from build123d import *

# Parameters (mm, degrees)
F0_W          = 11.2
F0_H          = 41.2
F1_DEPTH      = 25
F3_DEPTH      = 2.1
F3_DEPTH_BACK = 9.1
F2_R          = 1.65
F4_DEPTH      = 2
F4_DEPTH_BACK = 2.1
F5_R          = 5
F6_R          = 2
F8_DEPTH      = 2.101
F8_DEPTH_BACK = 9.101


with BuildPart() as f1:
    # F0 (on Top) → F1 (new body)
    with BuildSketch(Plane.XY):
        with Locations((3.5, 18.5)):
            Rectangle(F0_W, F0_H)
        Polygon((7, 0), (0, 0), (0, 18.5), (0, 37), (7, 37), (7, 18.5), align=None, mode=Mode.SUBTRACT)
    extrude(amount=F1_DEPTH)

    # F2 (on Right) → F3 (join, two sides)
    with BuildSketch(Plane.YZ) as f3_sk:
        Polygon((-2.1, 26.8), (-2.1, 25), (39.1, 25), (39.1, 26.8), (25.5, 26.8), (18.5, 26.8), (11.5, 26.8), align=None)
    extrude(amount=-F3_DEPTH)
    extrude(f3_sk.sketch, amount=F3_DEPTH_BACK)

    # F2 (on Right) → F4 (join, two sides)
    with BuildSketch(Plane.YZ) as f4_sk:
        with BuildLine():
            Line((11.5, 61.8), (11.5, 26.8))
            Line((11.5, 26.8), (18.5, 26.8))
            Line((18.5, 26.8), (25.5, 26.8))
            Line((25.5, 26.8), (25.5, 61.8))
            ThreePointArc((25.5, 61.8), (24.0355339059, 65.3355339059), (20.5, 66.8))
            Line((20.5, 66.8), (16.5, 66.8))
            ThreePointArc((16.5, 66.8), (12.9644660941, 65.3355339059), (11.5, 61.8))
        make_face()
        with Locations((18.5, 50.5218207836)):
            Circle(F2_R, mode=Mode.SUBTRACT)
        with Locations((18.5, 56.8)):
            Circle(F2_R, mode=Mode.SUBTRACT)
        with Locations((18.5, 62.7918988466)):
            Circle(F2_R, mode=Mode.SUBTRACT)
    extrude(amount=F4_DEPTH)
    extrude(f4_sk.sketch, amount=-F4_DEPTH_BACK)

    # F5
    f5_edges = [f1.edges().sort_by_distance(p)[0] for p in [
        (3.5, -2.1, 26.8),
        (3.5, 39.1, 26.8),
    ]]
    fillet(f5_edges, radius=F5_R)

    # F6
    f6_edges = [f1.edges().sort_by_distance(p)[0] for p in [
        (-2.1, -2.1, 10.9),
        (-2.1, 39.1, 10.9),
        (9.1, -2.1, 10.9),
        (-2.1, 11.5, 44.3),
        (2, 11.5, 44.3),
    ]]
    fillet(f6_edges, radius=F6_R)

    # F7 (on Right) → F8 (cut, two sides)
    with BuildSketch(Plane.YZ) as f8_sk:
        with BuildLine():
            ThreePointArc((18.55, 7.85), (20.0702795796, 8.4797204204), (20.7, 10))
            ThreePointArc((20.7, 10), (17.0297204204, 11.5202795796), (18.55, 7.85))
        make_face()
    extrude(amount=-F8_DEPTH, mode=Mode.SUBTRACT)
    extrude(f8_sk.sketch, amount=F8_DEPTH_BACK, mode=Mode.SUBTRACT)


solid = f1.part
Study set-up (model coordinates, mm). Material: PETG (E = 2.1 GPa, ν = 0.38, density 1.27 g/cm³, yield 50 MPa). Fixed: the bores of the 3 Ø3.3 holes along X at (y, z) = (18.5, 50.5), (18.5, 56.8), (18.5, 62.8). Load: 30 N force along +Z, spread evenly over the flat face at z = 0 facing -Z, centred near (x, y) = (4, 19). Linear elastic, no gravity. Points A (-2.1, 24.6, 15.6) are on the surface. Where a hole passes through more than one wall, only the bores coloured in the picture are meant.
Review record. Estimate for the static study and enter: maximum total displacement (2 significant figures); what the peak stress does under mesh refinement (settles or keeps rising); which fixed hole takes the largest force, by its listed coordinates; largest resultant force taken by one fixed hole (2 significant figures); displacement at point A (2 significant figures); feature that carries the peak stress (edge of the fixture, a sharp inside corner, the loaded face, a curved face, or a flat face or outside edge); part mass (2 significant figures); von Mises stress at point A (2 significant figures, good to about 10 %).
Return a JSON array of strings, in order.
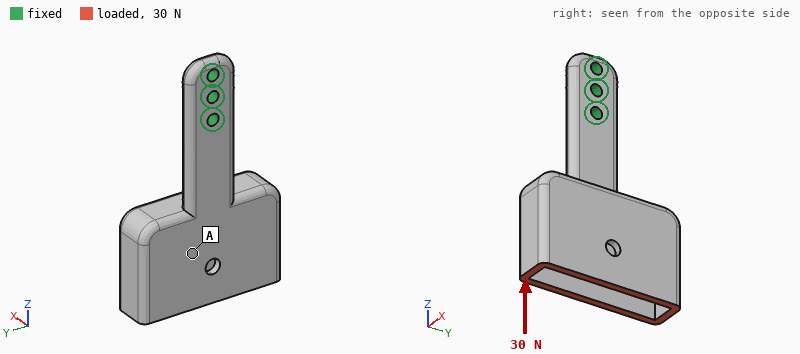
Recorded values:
["0.80 mm", "keeps rising", "(18.5, 50.5)", "24 N", "0.41 mm", "edge of the fixture", "9.6 g", "0.44 MPa"]
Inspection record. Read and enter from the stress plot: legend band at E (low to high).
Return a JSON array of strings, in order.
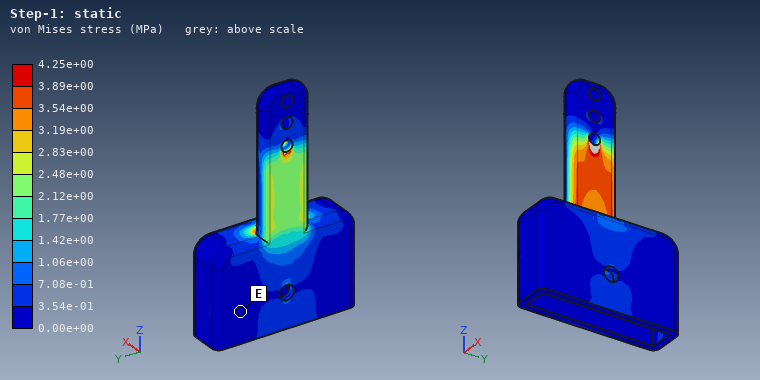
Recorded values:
["0.00e+00 to 3.54e-01 MPa"]
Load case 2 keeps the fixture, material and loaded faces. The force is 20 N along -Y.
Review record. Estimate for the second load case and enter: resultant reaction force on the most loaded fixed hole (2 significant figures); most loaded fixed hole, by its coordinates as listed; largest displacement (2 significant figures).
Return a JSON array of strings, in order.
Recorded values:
["86 N", "(18.5, 50.5)", "0.85 mm"]
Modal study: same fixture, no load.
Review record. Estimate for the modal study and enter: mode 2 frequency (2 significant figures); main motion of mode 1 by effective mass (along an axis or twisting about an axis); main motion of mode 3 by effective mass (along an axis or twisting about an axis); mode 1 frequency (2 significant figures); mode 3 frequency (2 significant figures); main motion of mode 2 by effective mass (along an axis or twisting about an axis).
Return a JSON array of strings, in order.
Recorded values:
["360 Hz", "along X", "along Y", "170 Hz", "460 Hz", "along Y"]
